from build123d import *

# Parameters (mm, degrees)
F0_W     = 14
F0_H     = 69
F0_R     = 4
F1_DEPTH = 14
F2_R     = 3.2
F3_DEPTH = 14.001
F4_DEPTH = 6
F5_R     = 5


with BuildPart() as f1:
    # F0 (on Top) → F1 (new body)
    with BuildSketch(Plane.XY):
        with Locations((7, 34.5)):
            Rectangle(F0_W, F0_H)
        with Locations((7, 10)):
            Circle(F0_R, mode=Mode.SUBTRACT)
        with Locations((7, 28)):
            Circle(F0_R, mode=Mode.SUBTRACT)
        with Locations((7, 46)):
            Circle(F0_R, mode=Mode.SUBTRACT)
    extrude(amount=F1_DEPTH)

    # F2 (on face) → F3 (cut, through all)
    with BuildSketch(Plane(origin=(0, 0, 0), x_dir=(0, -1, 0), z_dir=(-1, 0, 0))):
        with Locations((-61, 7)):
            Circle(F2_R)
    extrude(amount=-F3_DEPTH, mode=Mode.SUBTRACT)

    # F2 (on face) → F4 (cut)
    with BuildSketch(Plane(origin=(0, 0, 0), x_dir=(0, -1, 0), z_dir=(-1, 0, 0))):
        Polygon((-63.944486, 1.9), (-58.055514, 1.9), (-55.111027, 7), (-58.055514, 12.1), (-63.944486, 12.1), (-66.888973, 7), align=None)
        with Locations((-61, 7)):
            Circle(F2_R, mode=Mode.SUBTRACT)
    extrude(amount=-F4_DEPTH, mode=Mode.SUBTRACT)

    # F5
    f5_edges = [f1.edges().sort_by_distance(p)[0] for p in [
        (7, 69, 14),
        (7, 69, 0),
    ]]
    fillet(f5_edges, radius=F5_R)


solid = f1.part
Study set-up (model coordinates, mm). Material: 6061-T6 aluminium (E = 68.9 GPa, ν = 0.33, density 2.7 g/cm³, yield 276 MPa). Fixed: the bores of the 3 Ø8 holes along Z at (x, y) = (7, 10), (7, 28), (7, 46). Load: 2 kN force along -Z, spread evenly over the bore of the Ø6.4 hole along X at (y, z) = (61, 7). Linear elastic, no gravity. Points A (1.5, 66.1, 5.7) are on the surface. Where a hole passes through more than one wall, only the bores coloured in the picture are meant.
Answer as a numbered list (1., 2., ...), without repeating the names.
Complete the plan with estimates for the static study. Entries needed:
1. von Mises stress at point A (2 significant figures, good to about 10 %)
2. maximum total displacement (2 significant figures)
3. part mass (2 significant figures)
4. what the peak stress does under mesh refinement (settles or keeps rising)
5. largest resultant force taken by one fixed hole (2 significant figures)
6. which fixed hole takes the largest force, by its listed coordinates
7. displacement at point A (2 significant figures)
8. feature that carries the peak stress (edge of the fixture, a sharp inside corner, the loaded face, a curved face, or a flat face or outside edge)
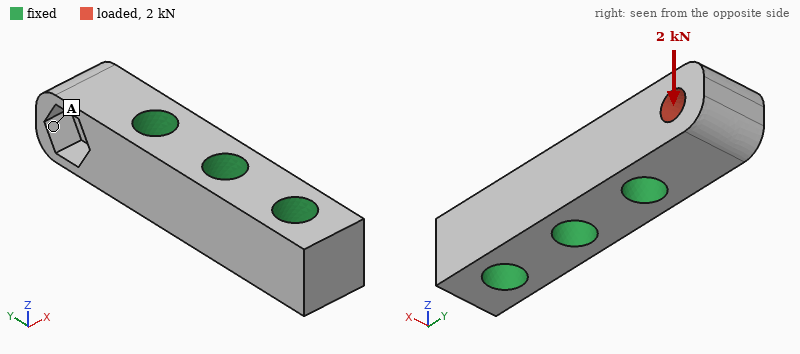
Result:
1. 11 MPa
2. 29 µm
3. 28 g
4. keeps rising
5. 2.0 kN
6. (7, 46)
7. 24 µm
8. edge of the fixture
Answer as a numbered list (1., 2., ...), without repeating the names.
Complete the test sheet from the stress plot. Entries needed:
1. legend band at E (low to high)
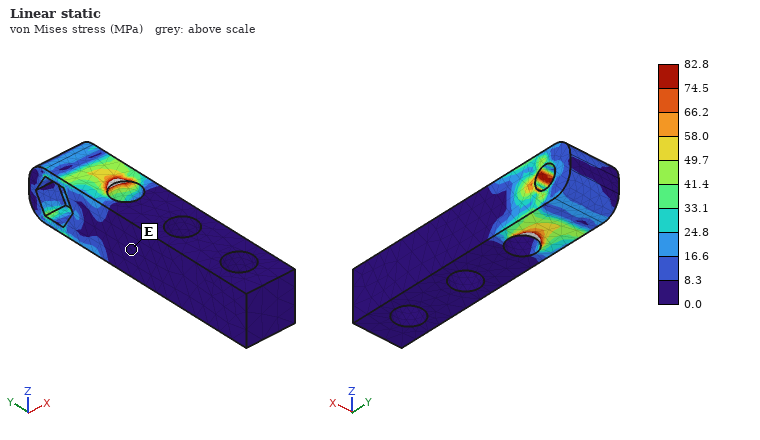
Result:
1. 0.0 to 8.3 MPa
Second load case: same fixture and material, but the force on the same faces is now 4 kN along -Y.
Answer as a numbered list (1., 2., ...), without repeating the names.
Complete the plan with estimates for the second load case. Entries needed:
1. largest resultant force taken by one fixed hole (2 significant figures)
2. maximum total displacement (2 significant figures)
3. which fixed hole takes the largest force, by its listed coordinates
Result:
1. 3.9 kN
2. 19 µm
3. (7, 46)
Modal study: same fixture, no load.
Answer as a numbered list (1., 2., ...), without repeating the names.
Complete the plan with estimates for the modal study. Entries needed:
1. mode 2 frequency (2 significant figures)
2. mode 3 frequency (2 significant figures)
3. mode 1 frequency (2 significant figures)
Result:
1. 20 kHz
2. 33 kHz
3. 19 kHz
